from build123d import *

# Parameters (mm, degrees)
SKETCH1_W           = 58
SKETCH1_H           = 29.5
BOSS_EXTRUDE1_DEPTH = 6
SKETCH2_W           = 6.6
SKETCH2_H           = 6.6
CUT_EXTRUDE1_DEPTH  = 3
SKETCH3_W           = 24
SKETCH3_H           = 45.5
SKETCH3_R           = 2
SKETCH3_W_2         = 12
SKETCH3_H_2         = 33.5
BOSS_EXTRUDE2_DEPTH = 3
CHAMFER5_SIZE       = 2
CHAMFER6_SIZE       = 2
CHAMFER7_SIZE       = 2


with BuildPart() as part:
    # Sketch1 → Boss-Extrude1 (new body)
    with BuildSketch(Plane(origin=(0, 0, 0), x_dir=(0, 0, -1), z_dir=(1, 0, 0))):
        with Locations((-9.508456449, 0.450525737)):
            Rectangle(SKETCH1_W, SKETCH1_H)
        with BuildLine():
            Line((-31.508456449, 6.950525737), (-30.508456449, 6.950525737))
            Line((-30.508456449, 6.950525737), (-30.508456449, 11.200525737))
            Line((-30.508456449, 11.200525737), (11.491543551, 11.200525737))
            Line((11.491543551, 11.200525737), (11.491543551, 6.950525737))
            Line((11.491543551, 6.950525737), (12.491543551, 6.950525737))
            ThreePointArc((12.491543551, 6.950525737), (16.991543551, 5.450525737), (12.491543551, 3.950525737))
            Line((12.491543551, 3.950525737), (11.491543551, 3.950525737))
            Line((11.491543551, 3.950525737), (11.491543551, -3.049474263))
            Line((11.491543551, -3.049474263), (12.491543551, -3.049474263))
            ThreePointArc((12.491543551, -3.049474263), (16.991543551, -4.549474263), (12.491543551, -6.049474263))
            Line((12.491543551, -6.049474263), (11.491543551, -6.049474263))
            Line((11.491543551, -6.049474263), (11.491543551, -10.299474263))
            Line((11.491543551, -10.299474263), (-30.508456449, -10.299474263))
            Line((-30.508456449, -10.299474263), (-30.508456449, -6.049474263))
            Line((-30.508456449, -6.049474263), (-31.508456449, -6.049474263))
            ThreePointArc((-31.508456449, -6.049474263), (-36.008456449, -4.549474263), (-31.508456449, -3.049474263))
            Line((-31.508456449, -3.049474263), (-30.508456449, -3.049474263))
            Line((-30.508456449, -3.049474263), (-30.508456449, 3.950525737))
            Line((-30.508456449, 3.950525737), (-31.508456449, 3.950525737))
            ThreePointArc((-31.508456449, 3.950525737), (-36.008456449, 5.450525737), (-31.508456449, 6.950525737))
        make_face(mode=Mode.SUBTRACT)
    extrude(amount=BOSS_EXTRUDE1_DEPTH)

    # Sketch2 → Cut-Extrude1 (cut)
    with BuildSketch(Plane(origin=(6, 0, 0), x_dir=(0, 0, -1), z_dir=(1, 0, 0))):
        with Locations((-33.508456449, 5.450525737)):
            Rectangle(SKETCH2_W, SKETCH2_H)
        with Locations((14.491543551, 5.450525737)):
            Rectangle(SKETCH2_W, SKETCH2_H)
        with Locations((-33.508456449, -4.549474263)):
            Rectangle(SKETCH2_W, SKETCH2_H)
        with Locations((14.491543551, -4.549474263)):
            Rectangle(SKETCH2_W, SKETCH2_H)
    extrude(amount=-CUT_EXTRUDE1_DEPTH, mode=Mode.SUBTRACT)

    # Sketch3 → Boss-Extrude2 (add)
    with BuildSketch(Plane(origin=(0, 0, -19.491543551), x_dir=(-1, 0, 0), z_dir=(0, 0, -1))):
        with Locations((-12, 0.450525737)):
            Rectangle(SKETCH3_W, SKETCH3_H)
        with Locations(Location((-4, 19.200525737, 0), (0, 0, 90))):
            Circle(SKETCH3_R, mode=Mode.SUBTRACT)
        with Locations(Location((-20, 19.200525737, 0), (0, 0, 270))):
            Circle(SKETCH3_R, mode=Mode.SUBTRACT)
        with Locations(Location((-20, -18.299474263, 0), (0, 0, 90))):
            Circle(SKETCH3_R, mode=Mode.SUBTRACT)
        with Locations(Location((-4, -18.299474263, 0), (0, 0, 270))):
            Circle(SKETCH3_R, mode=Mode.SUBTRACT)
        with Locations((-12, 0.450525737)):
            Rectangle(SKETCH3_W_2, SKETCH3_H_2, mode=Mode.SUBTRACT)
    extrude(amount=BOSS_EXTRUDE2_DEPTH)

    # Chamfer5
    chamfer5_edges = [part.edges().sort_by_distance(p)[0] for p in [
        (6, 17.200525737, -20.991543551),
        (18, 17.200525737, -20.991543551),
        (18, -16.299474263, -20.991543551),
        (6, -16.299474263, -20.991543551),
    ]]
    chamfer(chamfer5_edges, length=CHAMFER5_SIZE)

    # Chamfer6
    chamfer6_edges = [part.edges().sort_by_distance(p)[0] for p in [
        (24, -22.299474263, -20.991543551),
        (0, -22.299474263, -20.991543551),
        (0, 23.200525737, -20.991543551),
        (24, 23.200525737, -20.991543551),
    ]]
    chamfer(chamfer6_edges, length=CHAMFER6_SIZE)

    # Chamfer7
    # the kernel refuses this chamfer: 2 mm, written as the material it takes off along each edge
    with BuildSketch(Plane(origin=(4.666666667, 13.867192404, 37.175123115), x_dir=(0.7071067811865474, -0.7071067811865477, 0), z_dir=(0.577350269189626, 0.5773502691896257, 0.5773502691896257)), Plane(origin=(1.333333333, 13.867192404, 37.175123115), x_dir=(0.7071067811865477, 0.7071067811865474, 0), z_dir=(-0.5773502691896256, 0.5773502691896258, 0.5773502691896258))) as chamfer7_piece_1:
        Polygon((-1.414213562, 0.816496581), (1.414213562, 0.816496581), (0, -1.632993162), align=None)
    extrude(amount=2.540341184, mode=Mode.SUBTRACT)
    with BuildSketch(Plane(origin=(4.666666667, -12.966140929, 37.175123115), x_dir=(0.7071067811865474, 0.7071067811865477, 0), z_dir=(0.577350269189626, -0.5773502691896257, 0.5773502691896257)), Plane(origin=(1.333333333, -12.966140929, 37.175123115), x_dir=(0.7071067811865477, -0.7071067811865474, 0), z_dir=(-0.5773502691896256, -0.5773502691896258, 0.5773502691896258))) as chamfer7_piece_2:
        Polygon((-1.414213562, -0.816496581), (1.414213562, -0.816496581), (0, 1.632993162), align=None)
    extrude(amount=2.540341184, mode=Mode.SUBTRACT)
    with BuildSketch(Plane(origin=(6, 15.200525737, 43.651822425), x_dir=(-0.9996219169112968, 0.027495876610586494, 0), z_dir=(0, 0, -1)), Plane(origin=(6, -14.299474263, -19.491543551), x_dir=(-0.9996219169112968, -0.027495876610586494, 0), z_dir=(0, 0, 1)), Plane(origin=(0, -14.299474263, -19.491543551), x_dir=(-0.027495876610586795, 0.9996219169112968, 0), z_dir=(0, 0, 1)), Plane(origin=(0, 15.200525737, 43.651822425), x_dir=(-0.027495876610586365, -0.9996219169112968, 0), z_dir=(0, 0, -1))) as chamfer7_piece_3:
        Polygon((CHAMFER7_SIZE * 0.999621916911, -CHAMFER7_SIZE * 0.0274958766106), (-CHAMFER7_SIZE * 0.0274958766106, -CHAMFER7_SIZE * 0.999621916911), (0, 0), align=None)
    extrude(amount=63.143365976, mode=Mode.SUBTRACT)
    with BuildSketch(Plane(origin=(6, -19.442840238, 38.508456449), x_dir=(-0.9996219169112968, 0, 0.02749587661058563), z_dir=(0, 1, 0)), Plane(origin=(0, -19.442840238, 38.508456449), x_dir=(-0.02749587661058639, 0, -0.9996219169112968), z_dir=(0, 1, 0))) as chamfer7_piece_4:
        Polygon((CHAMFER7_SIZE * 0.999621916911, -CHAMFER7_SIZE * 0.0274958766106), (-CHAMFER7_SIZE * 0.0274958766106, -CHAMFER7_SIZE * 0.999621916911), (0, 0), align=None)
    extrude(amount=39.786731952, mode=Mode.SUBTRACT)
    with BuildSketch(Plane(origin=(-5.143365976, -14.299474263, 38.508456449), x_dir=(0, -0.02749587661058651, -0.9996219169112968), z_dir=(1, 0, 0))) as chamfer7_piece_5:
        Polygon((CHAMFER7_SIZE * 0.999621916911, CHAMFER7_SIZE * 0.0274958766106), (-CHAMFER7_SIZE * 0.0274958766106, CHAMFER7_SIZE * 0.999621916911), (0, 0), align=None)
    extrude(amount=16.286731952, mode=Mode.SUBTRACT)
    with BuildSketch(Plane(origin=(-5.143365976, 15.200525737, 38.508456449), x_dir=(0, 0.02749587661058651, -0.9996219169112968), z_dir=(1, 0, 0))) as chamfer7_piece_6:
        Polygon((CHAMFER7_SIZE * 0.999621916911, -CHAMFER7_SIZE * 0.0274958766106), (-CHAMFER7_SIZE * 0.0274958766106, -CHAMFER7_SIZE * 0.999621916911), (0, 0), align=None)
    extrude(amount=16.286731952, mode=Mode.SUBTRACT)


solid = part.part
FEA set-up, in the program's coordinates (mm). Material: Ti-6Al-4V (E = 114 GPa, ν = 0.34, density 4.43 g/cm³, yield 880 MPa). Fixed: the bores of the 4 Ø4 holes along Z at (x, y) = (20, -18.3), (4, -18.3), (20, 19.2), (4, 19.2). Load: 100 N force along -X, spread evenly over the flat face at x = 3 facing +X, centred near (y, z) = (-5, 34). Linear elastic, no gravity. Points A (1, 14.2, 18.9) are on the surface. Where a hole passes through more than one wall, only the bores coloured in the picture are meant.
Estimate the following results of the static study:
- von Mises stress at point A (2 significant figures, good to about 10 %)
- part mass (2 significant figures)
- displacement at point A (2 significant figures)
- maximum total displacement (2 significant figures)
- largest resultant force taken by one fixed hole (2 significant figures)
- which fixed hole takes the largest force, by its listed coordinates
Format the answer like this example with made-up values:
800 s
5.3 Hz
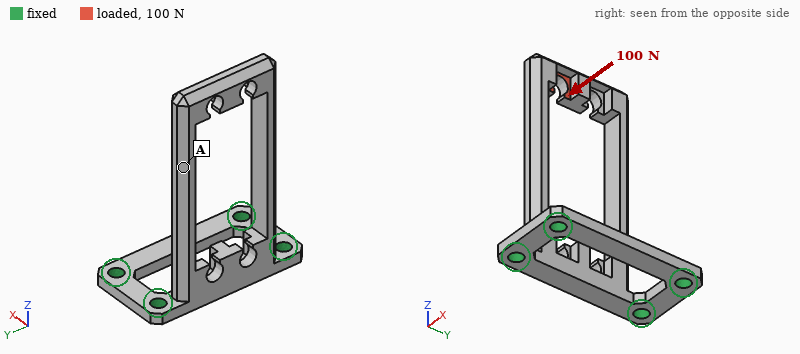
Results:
35 MPa
24 g
0.42 mm
0.83 mm
63 N
(4, -18.3)
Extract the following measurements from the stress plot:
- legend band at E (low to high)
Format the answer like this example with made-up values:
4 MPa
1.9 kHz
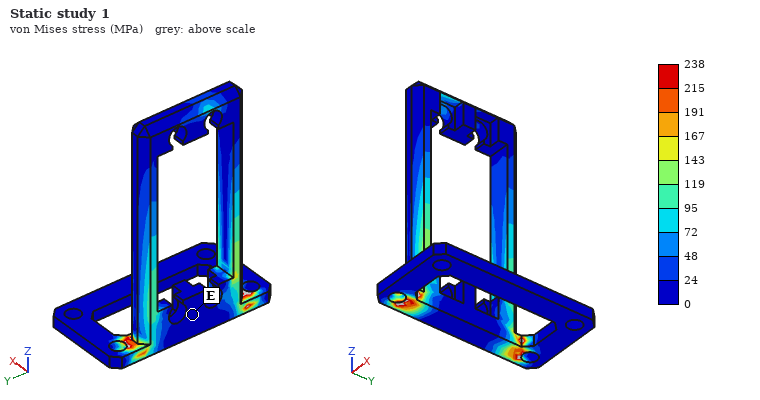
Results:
0 to 24 MPa
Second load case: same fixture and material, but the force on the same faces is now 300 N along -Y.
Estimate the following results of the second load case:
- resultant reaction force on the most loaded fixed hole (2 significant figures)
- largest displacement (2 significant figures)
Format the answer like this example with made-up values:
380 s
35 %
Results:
550 N
0.92 mm
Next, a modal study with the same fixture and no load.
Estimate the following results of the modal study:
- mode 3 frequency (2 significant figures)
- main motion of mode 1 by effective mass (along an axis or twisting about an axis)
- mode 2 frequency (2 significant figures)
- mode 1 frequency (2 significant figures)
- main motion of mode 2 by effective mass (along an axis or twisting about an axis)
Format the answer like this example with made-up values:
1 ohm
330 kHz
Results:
2400 Hz
along X
1300 Hz
780 Hz
along Y
